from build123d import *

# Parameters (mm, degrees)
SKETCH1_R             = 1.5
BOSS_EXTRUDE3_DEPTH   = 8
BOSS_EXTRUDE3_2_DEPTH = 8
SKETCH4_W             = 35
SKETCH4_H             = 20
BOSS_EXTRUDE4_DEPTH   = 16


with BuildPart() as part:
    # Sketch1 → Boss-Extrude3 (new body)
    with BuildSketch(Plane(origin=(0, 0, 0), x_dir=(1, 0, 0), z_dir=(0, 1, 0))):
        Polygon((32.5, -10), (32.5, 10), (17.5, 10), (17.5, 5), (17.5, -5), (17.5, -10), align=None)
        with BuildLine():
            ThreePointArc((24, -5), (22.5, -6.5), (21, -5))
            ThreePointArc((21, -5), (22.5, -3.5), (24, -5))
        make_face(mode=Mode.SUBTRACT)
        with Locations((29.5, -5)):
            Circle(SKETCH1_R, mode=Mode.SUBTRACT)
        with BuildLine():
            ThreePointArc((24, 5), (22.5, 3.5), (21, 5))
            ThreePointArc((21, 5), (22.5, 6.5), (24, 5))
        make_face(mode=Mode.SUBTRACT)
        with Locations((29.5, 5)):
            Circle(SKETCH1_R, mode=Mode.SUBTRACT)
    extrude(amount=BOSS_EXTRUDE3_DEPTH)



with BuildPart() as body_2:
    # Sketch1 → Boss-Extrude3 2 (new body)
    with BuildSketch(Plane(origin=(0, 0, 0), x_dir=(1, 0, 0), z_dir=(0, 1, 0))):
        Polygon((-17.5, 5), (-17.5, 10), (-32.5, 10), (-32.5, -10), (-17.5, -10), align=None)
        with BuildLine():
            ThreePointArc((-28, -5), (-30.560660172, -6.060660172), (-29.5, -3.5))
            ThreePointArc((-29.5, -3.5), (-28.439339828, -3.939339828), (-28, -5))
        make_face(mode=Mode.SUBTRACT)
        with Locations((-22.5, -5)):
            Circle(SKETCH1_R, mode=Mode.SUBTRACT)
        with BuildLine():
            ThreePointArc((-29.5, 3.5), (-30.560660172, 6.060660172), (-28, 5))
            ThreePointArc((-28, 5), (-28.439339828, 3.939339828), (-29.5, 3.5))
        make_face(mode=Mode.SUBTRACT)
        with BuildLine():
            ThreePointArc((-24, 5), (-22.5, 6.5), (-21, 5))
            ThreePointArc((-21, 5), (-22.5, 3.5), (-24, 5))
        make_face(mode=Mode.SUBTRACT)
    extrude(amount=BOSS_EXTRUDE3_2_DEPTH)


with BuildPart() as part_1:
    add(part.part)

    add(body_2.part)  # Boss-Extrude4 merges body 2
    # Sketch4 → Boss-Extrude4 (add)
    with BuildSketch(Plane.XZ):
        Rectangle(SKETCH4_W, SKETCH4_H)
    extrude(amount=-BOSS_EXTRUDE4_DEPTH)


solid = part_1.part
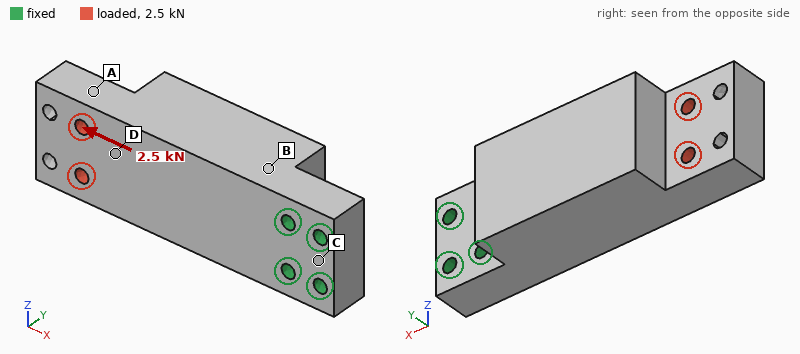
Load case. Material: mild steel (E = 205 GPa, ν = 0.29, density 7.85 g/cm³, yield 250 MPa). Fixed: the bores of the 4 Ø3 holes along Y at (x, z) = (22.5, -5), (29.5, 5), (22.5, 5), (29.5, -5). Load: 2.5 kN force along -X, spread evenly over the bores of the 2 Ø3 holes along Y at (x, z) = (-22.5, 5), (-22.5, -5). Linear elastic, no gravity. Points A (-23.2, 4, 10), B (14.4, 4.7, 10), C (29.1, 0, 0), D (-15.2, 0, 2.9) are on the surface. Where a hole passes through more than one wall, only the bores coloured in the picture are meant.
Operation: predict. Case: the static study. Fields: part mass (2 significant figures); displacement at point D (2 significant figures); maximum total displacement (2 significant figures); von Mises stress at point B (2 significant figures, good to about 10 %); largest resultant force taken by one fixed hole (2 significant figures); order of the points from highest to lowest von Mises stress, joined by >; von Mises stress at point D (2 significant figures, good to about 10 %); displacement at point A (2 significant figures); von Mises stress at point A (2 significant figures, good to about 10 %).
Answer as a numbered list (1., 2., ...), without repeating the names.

1. 120 g
2. 5.0 µm
3. 8.6 µm
4. 13 MPa
5. 1.1 kN
6. D > B > A > C
7. 19 MPa
8. 6.1 µm
9. 6.7 MPa
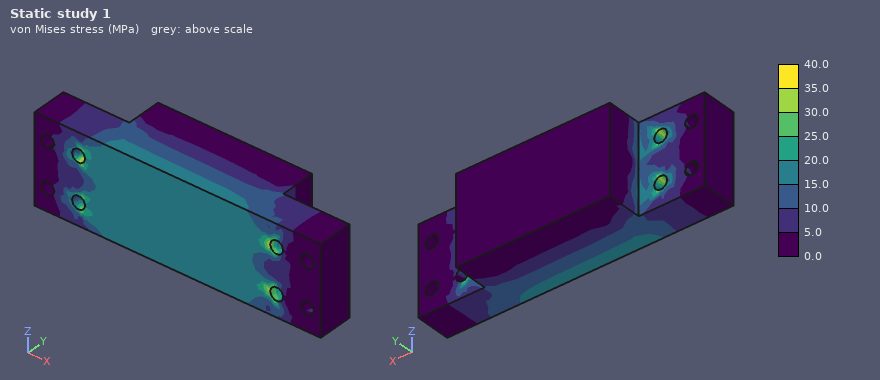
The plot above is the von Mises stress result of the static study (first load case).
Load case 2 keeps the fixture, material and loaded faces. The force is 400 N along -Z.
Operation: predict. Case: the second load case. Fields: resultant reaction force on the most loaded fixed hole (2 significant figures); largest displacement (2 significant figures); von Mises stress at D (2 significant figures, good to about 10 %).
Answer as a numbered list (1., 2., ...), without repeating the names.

1. 1.2 kN
2. 15 µm
3. 5.1 MPa
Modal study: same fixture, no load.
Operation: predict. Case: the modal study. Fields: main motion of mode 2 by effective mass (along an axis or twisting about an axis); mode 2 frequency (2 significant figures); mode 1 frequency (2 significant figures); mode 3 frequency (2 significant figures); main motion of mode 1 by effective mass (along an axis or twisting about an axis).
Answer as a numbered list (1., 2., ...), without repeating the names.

1. along Z
2. 4700 Hz
3. 2500 Hz
4. 11 kHz
5. along Y
